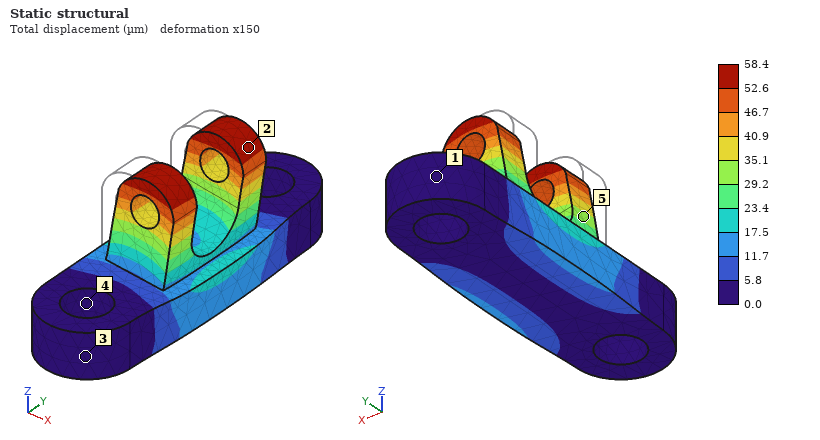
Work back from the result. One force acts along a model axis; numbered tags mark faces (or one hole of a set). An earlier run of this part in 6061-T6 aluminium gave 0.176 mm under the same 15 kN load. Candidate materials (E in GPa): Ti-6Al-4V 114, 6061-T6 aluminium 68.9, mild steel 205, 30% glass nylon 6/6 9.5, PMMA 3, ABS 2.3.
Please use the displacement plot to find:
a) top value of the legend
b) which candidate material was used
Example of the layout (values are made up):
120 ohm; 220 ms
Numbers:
58.4 µm; mild steel
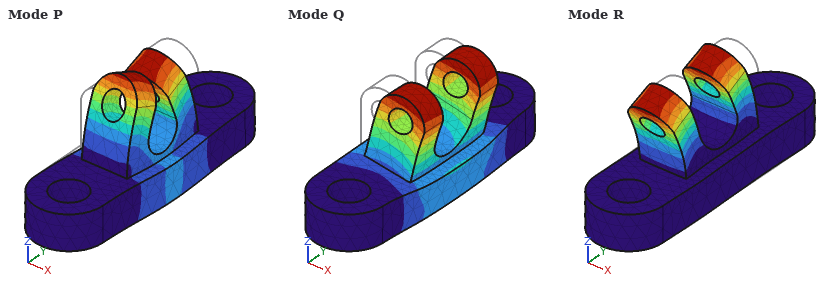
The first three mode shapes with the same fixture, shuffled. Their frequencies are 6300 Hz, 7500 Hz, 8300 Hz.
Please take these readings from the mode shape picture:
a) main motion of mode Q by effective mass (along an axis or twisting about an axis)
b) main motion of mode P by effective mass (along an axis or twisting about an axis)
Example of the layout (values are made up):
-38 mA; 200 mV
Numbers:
along X; along Z
